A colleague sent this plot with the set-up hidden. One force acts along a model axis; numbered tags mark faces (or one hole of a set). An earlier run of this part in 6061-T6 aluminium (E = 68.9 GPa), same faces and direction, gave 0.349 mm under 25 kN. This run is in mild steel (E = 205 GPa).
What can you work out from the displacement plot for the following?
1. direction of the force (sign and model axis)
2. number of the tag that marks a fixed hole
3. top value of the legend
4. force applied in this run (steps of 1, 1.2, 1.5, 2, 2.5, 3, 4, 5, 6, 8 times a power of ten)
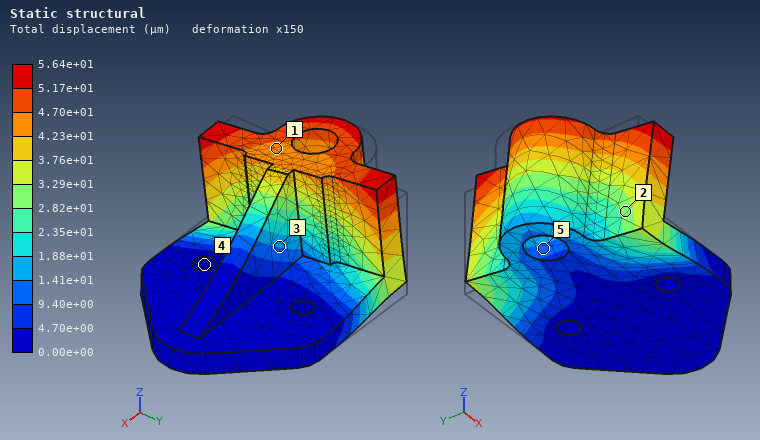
-Y
4
5.64e+01 µm
12 kN
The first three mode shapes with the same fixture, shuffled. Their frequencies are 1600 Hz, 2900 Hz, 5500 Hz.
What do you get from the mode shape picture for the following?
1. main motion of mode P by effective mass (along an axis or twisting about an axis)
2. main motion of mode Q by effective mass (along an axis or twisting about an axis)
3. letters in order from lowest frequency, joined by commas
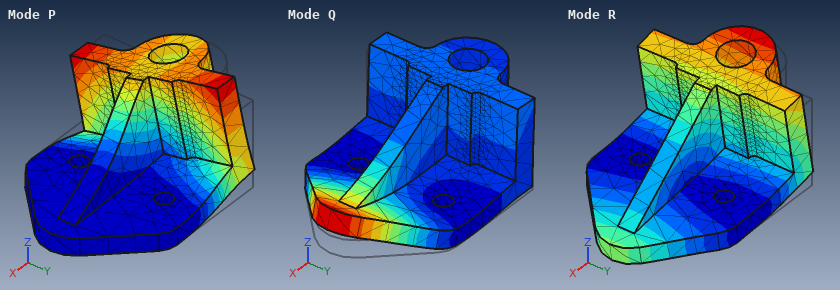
along Y
along Z
R, P, Q
